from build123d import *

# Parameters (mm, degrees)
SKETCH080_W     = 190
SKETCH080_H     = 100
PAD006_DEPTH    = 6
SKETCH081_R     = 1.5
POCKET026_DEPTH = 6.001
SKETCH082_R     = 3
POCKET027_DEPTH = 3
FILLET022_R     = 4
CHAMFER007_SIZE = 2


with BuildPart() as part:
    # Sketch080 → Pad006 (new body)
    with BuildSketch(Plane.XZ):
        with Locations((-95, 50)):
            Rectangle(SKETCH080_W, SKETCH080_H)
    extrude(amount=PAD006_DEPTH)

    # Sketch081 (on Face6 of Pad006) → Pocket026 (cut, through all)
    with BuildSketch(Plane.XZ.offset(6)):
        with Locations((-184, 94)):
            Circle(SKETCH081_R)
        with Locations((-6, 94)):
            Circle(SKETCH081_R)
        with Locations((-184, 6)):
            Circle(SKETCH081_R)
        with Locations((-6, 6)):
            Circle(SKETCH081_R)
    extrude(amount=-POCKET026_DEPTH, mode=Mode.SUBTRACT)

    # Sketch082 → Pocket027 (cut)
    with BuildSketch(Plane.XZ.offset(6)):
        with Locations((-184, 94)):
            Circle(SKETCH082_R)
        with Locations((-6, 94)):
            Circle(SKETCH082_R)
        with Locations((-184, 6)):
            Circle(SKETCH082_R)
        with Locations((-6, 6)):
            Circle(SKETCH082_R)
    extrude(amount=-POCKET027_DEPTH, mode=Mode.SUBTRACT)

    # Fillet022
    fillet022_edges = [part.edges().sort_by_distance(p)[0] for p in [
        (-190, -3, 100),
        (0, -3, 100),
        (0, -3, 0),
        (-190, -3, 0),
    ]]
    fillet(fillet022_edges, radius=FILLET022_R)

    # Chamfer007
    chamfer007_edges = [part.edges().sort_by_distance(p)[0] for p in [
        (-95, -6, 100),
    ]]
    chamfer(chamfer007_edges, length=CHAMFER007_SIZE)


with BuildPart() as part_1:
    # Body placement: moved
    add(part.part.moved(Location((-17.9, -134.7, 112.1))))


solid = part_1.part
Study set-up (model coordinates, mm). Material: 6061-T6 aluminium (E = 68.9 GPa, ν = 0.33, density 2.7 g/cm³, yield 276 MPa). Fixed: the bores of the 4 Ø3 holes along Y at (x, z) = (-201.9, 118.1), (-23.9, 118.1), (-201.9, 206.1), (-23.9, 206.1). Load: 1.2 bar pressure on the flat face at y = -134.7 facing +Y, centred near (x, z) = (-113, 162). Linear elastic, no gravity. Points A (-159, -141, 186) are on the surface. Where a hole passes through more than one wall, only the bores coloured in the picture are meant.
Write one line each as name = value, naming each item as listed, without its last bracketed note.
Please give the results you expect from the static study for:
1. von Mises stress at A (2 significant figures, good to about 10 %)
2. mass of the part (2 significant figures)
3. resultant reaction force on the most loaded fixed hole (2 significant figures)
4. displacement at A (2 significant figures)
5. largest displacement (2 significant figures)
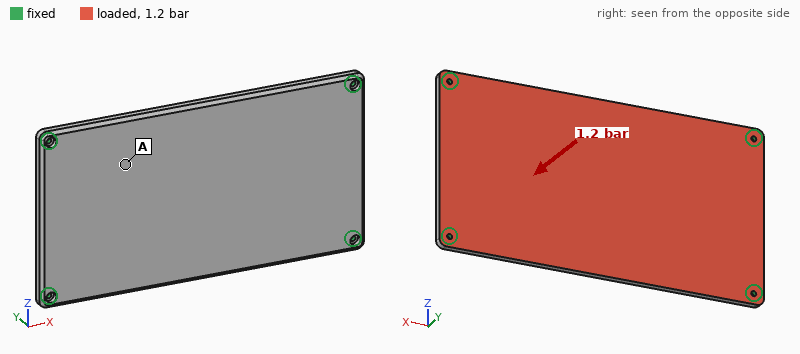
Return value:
von Mises stress at A = 27 MPa
mass of the part = 300 g
resultant reaction force on the most loaded fixed hole = 1.4 kN
displacement at A = 0.39 mm
largest displacement = 0.61 mm
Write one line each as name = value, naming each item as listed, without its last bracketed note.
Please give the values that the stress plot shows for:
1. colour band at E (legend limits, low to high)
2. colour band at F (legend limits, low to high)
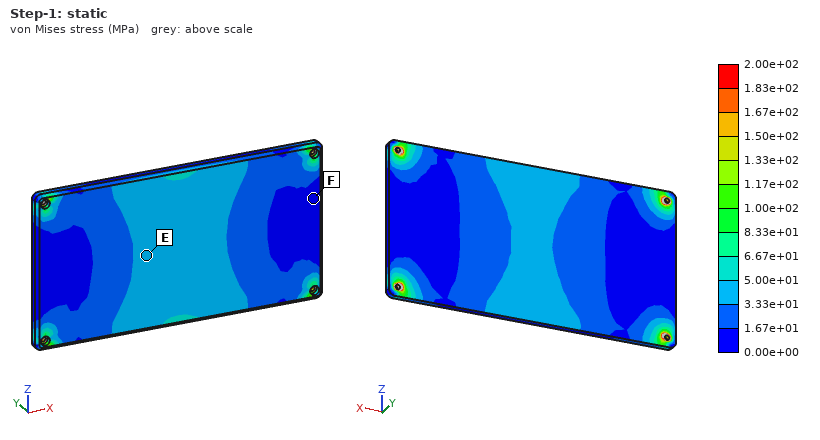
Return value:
colour band at E = 3.33e+01 to 5.00e+01 MPa
colour band at F = 0.00e+00 to 1.67e+01 MPa
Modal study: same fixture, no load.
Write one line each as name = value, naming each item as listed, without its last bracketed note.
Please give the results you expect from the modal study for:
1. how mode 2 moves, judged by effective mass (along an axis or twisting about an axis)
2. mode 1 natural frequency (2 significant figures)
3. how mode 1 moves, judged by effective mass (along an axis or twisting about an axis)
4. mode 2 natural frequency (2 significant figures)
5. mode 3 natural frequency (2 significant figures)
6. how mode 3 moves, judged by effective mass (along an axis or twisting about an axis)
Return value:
how mode 2 moves, judged by effective mass = twisting about X
mode 1 natural frequency = 640 Hz
how mode 1 moves, judged by effective mass = along Y
mode 2 natural frequency = 1300 Hz
mode 3 natural frequency = 1900 Hz
how mode 3 moves, judged by effective mass = twisting about Z
